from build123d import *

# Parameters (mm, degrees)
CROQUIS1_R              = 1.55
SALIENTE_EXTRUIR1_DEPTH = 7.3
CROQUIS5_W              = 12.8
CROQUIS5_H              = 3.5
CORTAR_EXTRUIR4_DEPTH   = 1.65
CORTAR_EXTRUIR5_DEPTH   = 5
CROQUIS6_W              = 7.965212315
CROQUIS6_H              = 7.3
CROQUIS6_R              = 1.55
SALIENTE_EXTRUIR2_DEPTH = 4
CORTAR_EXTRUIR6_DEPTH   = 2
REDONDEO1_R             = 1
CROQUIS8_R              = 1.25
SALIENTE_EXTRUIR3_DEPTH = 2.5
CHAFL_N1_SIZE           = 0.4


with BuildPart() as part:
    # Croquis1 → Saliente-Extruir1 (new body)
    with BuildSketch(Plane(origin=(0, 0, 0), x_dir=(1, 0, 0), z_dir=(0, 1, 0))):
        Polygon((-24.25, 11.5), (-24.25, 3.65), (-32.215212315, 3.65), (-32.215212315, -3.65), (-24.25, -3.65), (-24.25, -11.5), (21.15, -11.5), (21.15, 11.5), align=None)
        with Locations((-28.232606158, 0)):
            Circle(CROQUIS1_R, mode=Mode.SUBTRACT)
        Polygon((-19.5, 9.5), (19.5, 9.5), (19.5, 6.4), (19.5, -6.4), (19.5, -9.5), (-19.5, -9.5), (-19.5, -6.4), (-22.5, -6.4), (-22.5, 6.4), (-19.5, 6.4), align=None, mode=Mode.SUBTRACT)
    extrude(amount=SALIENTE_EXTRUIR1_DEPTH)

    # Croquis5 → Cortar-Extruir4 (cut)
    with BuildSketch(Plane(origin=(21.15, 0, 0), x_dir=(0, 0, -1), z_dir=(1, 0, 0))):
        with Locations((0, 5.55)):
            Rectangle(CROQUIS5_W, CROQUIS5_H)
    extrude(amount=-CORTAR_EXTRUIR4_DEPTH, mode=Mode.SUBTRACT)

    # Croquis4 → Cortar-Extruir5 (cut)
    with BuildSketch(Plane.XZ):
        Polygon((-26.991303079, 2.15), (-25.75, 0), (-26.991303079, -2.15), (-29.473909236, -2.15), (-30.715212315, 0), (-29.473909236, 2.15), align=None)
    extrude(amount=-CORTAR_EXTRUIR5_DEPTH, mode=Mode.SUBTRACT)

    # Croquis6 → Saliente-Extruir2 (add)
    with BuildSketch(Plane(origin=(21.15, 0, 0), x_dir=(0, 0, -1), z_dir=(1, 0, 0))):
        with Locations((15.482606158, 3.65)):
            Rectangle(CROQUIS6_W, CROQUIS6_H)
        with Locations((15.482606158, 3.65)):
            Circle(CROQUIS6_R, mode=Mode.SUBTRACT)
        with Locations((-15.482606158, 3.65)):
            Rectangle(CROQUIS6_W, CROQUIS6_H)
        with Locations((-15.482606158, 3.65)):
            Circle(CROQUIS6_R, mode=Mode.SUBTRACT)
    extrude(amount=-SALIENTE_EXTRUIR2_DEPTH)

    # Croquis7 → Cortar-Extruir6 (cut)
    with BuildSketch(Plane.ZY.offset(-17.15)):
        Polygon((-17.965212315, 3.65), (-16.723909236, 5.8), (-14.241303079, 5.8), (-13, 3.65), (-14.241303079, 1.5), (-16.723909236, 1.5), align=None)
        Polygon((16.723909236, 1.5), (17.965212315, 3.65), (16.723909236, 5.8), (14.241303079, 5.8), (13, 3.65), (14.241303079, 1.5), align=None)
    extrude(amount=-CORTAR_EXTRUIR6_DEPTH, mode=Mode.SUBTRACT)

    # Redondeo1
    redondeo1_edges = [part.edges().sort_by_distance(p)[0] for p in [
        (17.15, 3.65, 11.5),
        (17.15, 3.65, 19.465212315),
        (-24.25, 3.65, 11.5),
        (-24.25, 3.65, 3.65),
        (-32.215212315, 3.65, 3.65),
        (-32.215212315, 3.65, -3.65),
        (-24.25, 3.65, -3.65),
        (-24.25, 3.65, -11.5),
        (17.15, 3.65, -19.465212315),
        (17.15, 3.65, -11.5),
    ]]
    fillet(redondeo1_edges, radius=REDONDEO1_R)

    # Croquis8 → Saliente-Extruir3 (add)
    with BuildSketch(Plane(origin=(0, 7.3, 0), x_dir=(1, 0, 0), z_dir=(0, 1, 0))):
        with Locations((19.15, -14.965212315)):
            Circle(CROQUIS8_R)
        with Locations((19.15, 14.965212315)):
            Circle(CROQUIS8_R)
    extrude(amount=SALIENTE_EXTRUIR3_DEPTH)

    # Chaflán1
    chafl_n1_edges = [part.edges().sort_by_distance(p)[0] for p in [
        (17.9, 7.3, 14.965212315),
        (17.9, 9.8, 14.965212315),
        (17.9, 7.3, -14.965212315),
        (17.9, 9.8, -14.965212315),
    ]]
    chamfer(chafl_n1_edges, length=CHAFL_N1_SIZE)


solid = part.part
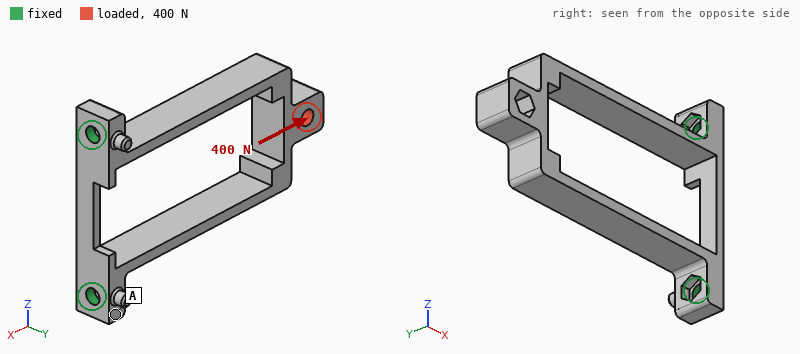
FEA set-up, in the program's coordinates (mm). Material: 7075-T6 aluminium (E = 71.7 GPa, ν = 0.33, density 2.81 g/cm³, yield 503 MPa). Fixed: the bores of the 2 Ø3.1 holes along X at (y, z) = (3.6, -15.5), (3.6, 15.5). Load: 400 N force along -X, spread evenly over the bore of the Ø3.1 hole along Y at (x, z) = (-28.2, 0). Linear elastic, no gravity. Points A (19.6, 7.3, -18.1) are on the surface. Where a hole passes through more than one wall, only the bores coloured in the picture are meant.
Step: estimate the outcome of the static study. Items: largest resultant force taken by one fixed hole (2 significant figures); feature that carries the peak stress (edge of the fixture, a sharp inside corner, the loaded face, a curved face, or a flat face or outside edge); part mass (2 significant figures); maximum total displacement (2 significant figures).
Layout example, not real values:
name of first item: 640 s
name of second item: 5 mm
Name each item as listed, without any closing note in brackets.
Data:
largest resultant force taken by one fixed hole: 200 N
feature that carries the peak stress: a curved face
part mass: 7.2 g
maximum total displacement: 0.25 mm
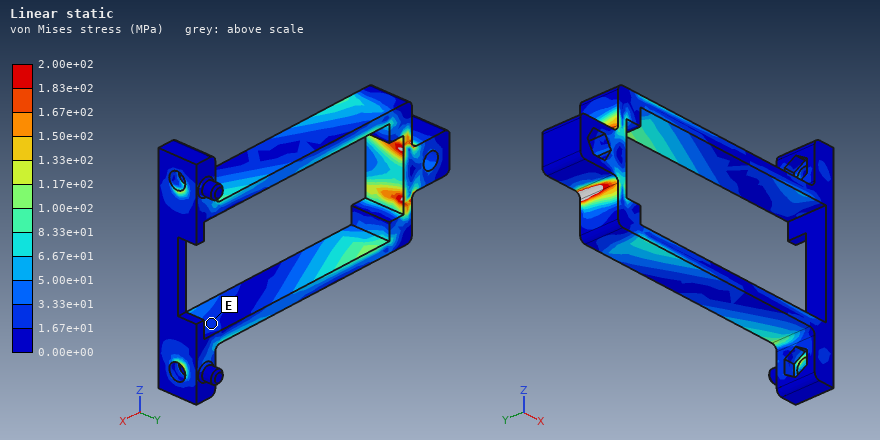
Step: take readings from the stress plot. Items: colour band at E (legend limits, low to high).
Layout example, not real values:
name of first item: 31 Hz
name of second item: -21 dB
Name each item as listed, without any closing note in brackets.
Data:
colour band at E: 1.67e+01 to 3.33e+01 MPa
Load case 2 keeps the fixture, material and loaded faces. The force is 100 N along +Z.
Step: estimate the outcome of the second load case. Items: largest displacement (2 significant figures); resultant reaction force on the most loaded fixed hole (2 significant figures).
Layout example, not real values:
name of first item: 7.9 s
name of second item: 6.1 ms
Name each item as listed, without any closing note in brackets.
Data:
largest displacement: 0.79 mm
resultant reaction force on the most loaded fixed hole: 140 N
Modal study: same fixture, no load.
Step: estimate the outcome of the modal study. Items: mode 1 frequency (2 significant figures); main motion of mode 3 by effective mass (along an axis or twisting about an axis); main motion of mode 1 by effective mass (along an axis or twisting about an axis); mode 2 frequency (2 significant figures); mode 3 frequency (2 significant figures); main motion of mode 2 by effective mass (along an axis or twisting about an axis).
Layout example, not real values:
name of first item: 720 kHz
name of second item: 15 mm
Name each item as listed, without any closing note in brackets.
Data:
mode 1 frequency: 980 Hz
main motion of mode 3 by effective mass: twisting about X
main motion of mode 1 by effective mass: along Z
mode 2 frequency: 1300 Hz
mode 3 frequency: 3000 Hz
main motion of mode 2 by effective mass: along Y
